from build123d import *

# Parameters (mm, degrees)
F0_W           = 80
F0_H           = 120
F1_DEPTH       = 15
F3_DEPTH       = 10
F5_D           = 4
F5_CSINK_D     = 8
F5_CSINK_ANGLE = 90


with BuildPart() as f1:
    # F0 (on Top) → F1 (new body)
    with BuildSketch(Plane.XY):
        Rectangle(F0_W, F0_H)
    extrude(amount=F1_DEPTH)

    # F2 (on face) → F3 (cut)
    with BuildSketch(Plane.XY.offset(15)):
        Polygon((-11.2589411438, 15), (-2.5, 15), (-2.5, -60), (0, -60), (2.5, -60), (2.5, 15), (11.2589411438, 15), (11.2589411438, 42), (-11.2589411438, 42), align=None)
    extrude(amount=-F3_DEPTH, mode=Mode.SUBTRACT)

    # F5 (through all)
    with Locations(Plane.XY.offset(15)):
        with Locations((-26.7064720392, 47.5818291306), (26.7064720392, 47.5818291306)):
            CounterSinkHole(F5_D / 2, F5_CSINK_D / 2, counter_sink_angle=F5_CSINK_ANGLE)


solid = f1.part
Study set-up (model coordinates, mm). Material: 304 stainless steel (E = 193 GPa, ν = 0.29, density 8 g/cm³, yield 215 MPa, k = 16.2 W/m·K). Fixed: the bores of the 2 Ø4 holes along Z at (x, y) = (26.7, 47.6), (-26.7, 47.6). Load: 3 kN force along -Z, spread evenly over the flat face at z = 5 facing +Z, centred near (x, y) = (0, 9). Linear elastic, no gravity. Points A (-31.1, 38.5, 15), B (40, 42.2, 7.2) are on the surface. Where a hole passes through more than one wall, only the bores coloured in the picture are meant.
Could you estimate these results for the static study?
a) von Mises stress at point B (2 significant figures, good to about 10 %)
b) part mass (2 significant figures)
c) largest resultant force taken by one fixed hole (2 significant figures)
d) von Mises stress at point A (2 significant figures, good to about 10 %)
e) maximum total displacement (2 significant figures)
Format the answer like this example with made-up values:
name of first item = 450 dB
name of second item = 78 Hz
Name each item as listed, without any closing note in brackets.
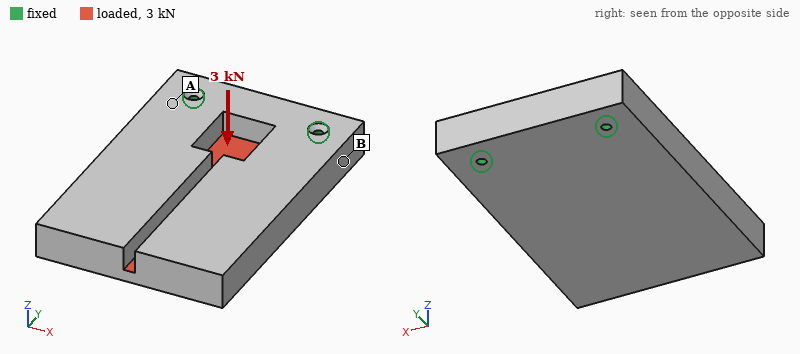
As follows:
von Mises stress at point B = 18 MPa
part mass = 1.1 kg
largest resultant force taken by one fixed hole = 1.5 kN
von Mises stress at point A = 39 MPa
maximum total displacement = 0.12 mm
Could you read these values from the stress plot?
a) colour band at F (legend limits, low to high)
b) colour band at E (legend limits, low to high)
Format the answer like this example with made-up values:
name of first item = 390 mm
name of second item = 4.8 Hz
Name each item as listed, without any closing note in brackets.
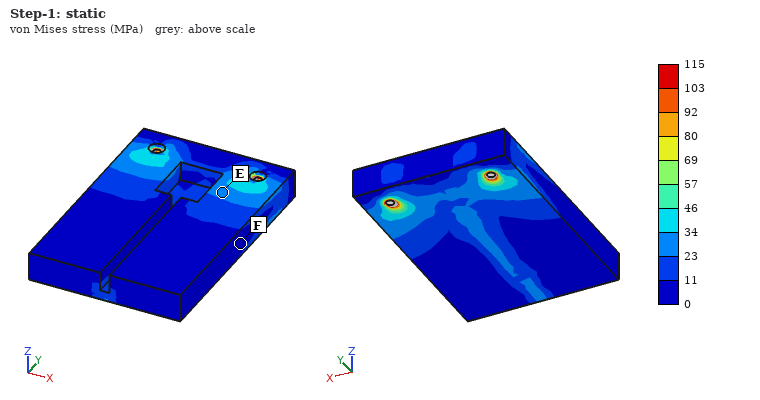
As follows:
colour band at F = 0 to 11 MPa
colour band at E = 23 to 34 MPa
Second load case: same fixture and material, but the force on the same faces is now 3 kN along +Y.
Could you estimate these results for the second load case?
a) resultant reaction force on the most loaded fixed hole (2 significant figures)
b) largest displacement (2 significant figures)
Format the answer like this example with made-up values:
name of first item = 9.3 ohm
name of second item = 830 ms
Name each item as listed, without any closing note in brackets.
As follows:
resultant reaction force on the most loaded fixed hole = 1.5 kN
largest displacement = 7.9 µm
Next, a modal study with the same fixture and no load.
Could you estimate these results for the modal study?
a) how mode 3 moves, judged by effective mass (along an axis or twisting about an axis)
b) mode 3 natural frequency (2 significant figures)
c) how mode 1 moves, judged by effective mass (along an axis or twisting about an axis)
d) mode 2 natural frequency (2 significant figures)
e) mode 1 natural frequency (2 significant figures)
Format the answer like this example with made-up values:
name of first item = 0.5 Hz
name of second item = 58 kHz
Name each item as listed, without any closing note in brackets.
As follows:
how mode 3 moves, judged by effective mass = along X
mode 3 natural frequency = 3400 Hz
how mode 1 moves, judged by effective mass = along Z
mode 2 natural frequency = 2400 Hz
mode 1 natural frequency = 820 Hz
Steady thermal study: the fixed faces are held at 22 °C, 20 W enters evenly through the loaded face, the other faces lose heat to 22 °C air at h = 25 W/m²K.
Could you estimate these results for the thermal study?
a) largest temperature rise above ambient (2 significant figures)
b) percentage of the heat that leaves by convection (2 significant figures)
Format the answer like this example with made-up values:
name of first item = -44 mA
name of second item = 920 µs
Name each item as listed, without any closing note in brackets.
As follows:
largest temperature rise above ambient = 35 K
percentage of the heat that leaves by convection = 50 %
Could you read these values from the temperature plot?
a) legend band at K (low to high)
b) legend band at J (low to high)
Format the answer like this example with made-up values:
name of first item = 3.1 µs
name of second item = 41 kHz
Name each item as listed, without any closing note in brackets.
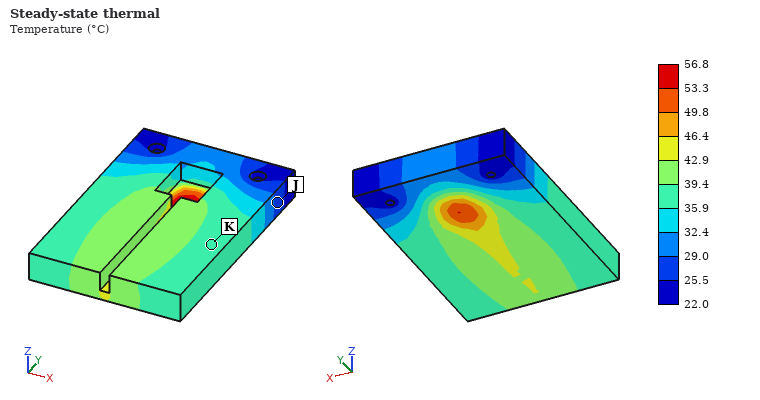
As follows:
legend band at K = 35.9 to 39.4 °C
legend band at J = 25.5 to 29.0 °C
